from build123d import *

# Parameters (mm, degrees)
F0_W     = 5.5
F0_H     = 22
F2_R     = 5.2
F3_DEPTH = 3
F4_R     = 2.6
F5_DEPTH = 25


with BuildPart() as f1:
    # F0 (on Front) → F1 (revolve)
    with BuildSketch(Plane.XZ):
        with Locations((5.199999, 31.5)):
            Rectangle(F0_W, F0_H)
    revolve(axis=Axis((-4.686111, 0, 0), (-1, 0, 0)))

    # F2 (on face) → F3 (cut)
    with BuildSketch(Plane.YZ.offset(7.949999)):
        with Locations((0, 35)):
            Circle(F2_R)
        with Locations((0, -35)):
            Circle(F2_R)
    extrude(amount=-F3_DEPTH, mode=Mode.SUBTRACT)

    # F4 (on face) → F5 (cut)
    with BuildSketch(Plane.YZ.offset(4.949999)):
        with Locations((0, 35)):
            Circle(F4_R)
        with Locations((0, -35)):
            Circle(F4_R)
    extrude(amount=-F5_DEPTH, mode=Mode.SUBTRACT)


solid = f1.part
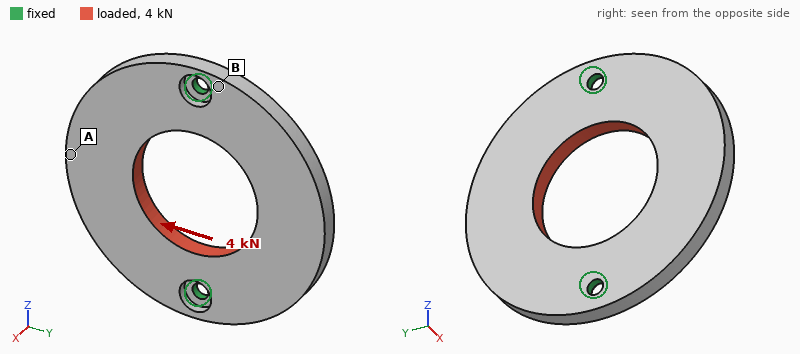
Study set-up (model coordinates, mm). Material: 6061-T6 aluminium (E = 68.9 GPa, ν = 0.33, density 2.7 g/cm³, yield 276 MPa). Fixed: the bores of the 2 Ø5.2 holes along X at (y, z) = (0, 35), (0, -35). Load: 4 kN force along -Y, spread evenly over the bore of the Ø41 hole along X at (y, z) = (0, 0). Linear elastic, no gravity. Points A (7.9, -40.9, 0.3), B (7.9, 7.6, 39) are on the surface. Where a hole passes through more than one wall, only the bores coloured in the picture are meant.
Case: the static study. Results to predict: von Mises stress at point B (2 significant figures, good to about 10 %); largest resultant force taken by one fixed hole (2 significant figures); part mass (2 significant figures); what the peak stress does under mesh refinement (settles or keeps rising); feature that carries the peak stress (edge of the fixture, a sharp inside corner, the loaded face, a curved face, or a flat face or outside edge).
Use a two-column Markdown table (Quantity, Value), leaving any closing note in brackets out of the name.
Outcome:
| Quantity | Value |
|---|---|
| von Mises stress at point B | 19 MPa |
| largest resultant force taken by one fixed hole | 2.0 kN |
| part mass | 63 g |
| what the peak stress does under mesh refinement | keeps rising |
| feature that carries the peak stress | edge of the fixture |
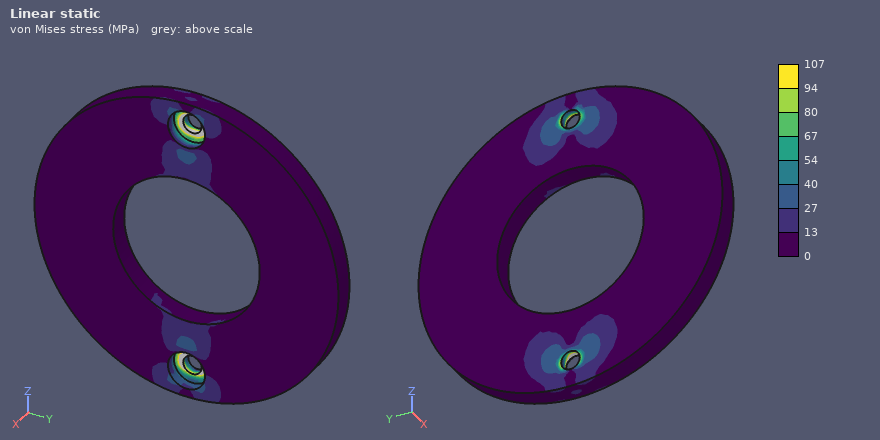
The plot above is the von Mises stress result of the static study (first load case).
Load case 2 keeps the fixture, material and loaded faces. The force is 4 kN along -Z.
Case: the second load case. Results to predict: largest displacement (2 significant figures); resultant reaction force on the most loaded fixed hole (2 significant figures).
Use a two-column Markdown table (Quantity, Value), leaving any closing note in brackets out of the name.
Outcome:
| Quantity | Value |
|---|---|
| largest displacement | 14 µm |
| resultant reaction force on the most loaded fixed hole | 2.0 kN |
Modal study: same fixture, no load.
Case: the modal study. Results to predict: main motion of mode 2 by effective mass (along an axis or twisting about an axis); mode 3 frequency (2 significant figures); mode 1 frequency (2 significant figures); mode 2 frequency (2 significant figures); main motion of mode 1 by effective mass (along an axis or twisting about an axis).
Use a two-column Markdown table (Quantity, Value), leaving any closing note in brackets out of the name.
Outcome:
| Quantity | Value |
|---|---|
| main motion of mode 2 by effective mass | along X |
| mode 3 frequency | 4300 Hz |
| mode 1 frequency | 1300 Hz |
| mode 2 frequency | 2000 Hz |
| main motion of mode 1 by effective mass | twisting about Z |
